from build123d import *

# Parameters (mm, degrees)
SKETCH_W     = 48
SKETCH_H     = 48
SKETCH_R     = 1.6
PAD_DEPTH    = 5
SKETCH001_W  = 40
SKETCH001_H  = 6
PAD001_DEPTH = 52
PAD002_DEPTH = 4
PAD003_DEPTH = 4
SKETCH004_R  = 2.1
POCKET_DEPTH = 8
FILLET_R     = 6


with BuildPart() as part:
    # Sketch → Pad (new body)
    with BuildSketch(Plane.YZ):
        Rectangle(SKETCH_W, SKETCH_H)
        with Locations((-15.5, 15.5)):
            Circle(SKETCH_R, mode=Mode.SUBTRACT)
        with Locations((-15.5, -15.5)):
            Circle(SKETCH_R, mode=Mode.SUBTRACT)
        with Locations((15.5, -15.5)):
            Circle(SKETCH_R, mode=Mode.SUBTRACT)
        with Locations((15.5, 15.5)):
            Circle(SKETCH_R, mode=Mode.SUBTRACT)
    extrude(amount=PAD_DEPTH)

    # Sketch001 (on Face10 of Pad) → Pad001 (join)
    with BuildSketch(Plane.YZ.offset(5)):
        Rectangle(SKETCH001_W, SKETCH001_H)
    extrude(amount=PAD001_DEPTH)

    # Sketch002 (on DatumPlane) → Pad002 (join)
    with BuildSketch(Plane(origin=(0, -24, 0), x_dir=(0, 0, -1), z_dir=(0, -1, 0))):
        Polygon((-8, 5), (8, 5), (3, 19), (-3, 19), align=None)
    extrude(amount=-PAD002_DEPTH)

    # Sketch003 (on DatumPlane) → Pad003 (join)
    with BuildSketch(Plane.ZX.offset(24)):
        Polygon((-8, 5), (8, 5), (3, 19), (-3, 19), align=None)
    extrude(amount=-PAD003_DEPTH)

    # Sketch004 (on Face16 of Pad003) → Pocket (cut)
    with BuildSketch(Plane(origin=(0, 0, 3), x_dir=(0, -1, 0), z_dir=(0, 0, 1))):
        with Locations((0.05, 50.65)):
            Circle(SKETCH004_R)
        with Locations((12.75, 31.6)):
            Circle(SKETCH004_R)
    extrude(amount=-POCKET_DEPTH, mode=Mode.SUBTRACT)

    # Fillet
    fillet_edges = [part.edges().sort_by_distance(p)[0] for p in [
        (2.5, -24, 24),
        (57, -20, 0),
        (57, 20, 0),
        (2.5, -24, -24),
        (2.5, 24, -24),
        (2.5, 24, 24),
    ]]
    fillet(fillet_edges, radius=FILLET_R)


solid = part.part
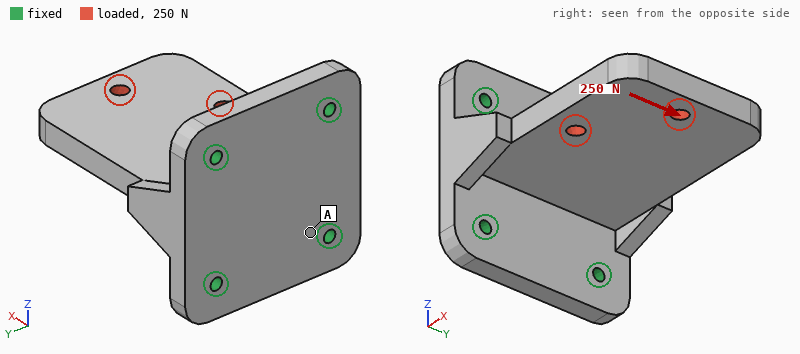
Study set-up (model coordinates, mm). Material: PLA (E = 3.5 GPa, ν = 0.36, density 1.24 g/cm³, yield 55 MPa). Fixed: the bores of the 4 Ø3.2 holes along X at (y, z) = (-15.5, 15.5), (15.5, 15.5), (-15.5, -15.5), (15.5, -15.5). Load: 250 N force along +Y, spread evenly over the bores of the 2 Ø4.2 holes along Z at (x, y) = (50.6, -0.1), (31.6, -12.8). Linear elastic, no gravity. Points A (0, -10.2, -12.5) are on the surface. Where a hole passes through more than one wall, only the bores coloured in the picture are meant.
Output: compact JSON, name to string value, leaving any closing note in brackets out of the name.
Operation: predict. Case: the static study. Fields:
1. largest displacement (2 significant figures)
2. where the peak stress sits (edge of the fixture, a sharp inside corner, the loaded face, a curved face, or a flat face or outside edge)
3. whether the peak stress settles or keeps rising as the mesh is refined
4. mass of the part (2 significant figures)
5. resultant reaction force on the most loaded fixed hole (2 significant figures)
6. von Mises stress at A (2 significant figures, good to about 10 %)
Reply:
{"largest displacement": "0.27 mm", "where the peak stress sits": "edge of the fixture", "whether the peak stress settles or keeps rising as the mesh is refined": "keeps rising", "mass of the part": "31 g", "resultant reaction force on the most loaded fixed hole": "160 N", "von Mises stress at A": "2.4 MPa"}
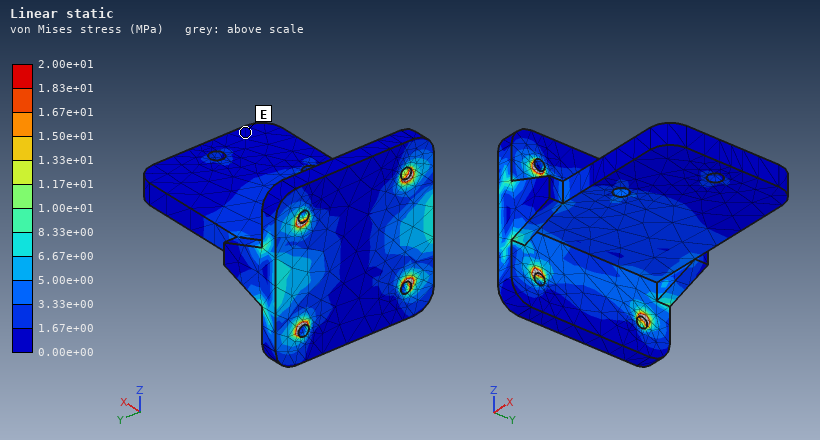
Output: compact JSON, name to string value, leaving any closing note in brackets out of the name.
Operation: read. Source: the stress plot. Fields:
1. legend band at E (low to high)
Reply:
{"legend band at E": "0.00e+00 to 1.67e+00 MPa"}
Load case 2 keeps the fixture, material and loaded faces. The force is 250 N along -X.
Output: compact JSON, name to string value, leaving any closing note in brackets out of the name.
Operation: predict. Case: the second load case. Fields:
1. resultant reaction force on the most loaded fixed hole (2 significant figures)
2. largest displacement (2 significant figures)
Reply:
{"resultant reaction force on the most loaded fixed hole": "87 N", "largest displacement": "63 µm"}
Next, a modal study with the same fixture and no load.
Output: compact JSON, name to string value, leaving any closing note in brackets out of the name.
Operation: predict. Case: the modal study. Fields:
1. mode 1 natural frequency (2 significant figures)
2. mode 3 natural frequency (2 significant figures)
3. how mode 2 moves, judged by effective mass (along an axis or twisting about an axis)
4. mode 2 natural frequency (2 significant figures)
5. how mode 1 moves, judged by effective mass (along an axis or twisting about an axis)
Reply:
{"mode 1 natural frequency": "640 Hz", "mode 3 natural frequency": "1900 Hz", "how mode 2 moves, judged by effective mass": "along Y", "mode 2 natural frequency": "1700 Hz", "how mode 1 moves, judged by effective mass": "along Z"}
